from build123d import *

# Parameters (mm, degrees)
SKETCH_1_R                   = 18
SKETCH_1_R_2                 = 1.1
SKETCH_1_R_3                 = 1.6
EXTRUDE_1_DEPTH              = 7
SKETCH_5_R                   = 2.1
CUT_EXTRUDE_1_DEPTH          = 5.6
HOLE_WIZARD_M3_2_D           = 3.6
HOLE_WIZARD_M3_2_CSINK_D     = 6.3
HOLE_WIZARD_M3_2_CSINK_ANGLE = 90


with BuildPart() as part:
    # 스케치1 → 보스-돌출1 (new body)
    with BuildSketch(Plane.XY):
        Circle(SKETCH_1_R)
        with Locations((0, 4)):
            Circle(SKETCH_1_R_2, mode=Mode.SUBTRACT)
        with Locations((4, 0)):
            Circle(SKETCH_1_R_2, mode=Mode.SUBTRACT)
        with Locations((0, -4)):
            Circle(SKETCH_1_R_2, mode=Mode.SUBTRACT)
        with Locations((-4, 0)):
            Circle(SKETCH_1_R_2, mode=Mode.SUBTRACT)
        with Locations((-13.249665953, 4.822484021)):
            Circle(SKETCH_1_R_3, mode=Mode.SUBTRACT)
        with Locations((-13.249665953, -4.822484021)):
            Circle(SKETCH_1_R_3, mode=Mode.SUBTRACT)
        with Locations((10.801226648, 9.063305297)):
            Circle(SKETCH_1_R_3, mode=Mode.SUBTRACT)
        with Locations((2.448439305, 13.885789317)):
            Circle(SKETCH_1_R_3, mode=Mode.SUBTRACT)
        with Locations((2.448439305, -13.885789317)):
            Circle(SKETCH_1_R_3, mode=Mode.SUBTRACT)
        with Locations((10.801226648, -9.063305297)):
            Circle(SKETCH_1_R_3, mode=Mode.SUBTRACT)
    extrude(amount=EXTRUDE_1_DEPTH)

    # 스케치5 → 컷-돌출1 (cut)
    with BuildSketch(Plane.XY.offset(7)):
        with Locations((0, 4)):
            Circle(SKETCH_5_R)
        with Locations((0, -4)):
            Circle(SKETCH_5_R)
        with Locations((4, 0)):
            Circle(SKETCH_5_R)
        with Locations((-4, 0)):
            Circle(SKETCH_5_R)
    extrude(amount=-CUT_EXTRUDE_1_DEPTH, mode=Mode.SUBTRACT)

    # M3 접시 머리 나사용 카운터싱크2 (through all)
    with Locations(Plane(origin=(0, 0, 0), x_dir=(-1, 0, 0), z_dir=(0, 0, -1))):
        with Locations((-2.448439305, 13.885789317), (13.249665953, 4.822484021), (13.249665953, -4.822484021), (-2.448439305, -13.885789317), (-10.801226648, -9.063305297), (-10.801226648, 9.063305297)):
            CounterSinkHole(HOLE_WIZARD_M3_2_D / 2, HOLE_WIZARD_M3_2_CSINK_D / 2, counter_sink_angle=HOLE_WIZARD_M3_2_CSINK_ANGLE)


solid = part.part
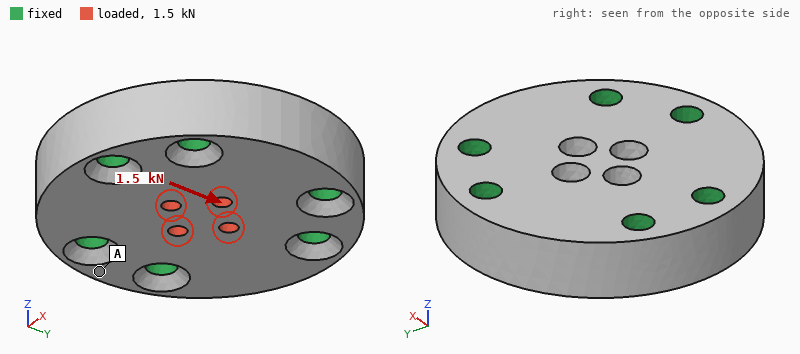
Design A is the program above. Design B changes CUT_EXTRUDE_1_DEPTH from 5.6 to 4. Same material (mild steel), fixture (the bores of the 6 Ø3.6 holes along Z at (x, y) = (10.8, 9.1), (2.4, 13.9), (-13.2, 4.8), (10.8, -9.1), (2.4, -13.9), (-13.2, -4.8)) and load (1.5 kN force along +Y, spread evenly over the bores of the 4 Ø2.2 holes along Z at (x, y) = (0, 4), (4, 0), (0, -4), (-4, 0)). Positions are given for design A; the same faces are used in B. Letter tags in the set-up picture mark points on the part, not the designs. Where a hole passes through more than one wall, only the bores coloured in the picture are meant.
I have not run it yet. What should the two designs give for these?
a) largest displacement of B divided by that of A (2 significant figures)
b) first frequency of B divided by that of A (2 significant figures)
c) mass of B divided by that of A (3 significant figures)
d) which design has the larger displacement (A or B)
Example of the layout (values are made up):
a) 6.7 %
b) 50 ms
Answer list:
a) 0.66
b) 0.98
c) 1.01
d) A
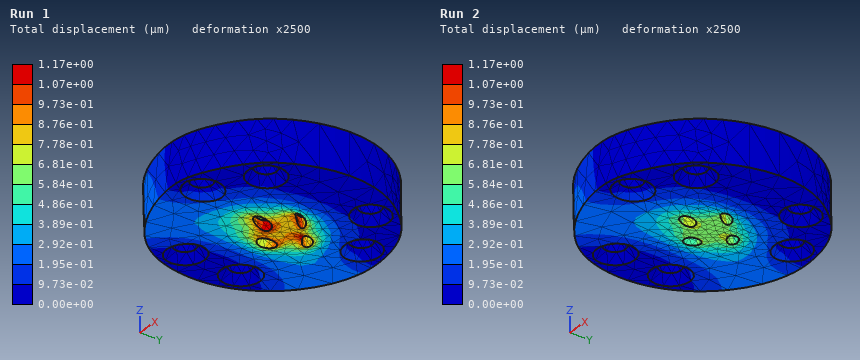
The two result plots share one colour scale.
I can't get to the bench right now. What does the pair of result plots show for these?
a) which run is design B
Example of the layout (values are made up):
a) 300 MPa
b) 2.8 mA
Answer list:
a) Run 2
